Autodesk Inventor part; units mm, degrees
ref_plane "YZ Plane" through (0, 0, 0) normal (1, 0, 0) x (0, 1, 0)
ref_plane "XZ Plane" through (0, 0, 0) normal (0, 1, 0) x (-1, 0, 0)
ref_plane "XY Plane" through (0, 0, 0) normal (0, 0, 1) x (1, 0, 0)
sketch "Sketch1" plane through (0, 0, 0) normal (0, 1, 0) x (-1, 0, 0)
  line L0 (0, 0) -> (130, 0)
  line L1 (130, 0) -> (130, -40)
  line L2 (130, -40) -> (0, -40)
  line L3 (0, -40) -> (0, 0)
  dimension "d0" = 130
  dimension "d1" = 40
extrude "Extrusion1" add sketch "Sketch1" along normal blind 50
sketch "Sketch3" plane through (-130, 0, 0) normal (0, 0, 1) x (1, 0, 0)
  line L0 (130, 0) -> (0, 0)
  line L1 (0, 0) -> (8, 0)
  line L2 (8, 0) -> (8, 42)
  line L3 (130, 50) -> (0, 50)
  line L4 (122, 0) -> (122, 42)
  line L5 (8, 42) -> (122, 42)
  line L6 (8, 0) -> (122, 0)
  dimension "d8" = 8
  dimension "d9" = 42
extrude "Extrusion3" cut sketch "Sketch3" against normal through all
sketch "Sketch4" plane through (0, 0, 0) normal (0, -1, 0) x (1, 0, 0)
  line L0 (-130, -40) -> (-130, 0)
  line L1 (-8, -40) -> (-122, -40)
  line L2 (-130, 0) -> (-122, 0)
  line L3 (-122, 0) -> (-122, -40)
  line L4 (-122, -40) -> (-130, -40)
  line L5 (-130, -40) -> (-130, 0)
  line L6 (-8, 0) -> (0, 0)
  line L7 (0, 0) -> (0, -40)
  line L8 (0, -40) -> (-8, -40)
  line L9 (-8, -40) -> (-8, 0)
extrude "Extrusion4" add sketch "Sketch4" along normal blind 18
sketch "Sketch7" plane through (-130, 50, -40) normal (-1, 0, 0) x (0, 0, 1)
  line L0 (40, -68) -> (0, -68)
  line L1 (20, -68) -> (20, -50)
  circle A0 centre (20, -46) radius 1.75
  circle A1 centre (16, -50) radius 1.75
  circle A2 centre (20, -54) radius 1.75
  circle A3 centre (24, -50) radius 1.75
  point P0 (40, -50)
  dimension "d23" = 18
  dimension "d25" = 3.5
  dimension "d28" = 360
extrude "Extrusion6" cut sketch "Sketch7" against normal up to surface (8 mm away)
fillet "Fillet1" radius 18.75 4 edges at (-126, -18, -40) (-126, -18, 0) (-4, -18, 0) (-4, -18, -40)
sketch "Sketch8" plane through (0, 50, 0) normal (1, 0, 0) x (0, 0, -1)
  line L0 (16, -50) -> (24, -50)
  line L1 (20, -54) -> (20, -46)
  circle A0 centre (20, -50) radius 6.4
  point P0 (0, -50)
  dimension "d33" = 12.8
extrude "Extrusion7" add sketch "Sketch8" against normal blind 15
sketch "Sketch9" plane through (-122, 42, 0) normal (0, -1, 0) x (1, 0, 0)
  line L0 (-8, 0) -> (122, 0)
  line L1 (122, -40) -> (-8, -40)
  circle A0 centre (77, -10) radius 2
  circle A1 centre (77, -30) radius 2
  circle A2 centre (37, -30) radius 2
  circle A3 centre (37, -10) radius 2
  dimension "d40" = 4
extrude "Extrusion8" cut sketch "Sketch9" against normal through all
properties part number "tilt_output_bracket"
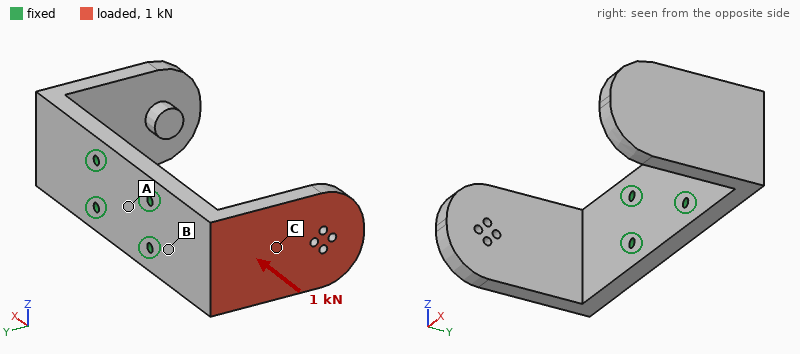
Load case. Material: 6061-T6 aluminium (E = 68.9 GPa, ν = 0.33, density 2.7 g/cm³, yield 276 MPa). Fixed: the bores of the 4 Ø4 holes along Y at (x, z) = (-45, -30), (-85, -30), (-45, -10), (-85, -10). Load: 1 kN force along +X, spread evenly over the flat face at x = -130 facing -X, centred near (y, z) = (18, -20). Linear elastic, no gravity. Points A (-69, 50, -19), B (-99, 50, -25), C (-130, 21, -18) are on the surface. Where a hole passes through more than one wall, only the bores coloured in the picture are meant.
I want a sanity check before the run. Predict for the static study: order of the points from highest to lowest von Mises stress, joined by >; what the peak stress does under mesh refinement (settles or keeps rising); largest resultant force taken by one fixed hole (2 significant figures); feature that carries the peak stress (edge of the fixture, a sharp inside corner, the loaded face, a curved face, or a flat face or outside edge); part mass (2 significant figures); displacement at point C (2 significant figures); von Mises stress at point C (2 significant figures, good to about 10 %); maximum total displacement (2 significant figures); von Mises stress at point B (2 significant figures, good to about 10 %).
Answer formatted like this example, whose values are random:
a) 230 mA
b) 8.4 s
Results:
a) B > C > A
b) keeps rising
c) 460 N
d) edge of the fixture
e) 210 g
f) 0.38 mm
g) 20 MPa
h) 0.84 mm
i) 56 MPa
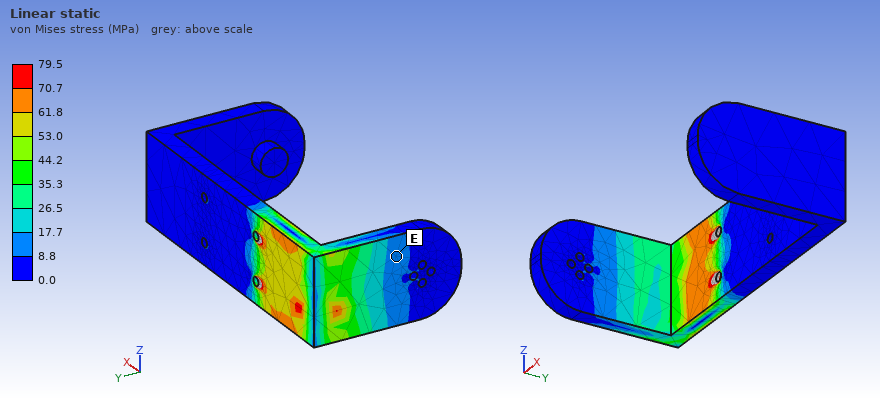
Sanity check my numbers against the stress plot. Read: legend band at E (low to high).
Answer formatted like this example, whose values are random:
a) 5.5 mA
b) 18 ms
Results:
a) 8.8 to 17.7 MPa
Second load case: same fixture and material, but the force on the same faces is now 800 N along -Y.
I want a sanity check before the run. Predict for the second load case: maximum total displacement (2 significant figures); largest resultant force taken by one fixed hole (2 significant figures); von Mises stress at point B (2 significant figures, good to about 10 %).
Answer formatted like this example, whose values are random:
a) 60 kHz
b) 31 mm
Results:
a) 0.52 mm
b) 500 N
c) 53 MPa
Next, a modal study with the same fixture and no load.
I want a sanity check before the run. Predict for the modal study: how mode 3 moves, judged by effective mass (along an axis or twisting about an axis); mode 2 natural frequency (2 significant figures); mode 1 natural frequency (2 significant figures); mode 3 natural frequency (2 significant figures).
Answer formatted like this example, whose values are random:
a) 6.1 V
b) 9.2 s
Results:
a) along Z
b) 840 Hz
c) 810 Hz
d) 1300 Hz
